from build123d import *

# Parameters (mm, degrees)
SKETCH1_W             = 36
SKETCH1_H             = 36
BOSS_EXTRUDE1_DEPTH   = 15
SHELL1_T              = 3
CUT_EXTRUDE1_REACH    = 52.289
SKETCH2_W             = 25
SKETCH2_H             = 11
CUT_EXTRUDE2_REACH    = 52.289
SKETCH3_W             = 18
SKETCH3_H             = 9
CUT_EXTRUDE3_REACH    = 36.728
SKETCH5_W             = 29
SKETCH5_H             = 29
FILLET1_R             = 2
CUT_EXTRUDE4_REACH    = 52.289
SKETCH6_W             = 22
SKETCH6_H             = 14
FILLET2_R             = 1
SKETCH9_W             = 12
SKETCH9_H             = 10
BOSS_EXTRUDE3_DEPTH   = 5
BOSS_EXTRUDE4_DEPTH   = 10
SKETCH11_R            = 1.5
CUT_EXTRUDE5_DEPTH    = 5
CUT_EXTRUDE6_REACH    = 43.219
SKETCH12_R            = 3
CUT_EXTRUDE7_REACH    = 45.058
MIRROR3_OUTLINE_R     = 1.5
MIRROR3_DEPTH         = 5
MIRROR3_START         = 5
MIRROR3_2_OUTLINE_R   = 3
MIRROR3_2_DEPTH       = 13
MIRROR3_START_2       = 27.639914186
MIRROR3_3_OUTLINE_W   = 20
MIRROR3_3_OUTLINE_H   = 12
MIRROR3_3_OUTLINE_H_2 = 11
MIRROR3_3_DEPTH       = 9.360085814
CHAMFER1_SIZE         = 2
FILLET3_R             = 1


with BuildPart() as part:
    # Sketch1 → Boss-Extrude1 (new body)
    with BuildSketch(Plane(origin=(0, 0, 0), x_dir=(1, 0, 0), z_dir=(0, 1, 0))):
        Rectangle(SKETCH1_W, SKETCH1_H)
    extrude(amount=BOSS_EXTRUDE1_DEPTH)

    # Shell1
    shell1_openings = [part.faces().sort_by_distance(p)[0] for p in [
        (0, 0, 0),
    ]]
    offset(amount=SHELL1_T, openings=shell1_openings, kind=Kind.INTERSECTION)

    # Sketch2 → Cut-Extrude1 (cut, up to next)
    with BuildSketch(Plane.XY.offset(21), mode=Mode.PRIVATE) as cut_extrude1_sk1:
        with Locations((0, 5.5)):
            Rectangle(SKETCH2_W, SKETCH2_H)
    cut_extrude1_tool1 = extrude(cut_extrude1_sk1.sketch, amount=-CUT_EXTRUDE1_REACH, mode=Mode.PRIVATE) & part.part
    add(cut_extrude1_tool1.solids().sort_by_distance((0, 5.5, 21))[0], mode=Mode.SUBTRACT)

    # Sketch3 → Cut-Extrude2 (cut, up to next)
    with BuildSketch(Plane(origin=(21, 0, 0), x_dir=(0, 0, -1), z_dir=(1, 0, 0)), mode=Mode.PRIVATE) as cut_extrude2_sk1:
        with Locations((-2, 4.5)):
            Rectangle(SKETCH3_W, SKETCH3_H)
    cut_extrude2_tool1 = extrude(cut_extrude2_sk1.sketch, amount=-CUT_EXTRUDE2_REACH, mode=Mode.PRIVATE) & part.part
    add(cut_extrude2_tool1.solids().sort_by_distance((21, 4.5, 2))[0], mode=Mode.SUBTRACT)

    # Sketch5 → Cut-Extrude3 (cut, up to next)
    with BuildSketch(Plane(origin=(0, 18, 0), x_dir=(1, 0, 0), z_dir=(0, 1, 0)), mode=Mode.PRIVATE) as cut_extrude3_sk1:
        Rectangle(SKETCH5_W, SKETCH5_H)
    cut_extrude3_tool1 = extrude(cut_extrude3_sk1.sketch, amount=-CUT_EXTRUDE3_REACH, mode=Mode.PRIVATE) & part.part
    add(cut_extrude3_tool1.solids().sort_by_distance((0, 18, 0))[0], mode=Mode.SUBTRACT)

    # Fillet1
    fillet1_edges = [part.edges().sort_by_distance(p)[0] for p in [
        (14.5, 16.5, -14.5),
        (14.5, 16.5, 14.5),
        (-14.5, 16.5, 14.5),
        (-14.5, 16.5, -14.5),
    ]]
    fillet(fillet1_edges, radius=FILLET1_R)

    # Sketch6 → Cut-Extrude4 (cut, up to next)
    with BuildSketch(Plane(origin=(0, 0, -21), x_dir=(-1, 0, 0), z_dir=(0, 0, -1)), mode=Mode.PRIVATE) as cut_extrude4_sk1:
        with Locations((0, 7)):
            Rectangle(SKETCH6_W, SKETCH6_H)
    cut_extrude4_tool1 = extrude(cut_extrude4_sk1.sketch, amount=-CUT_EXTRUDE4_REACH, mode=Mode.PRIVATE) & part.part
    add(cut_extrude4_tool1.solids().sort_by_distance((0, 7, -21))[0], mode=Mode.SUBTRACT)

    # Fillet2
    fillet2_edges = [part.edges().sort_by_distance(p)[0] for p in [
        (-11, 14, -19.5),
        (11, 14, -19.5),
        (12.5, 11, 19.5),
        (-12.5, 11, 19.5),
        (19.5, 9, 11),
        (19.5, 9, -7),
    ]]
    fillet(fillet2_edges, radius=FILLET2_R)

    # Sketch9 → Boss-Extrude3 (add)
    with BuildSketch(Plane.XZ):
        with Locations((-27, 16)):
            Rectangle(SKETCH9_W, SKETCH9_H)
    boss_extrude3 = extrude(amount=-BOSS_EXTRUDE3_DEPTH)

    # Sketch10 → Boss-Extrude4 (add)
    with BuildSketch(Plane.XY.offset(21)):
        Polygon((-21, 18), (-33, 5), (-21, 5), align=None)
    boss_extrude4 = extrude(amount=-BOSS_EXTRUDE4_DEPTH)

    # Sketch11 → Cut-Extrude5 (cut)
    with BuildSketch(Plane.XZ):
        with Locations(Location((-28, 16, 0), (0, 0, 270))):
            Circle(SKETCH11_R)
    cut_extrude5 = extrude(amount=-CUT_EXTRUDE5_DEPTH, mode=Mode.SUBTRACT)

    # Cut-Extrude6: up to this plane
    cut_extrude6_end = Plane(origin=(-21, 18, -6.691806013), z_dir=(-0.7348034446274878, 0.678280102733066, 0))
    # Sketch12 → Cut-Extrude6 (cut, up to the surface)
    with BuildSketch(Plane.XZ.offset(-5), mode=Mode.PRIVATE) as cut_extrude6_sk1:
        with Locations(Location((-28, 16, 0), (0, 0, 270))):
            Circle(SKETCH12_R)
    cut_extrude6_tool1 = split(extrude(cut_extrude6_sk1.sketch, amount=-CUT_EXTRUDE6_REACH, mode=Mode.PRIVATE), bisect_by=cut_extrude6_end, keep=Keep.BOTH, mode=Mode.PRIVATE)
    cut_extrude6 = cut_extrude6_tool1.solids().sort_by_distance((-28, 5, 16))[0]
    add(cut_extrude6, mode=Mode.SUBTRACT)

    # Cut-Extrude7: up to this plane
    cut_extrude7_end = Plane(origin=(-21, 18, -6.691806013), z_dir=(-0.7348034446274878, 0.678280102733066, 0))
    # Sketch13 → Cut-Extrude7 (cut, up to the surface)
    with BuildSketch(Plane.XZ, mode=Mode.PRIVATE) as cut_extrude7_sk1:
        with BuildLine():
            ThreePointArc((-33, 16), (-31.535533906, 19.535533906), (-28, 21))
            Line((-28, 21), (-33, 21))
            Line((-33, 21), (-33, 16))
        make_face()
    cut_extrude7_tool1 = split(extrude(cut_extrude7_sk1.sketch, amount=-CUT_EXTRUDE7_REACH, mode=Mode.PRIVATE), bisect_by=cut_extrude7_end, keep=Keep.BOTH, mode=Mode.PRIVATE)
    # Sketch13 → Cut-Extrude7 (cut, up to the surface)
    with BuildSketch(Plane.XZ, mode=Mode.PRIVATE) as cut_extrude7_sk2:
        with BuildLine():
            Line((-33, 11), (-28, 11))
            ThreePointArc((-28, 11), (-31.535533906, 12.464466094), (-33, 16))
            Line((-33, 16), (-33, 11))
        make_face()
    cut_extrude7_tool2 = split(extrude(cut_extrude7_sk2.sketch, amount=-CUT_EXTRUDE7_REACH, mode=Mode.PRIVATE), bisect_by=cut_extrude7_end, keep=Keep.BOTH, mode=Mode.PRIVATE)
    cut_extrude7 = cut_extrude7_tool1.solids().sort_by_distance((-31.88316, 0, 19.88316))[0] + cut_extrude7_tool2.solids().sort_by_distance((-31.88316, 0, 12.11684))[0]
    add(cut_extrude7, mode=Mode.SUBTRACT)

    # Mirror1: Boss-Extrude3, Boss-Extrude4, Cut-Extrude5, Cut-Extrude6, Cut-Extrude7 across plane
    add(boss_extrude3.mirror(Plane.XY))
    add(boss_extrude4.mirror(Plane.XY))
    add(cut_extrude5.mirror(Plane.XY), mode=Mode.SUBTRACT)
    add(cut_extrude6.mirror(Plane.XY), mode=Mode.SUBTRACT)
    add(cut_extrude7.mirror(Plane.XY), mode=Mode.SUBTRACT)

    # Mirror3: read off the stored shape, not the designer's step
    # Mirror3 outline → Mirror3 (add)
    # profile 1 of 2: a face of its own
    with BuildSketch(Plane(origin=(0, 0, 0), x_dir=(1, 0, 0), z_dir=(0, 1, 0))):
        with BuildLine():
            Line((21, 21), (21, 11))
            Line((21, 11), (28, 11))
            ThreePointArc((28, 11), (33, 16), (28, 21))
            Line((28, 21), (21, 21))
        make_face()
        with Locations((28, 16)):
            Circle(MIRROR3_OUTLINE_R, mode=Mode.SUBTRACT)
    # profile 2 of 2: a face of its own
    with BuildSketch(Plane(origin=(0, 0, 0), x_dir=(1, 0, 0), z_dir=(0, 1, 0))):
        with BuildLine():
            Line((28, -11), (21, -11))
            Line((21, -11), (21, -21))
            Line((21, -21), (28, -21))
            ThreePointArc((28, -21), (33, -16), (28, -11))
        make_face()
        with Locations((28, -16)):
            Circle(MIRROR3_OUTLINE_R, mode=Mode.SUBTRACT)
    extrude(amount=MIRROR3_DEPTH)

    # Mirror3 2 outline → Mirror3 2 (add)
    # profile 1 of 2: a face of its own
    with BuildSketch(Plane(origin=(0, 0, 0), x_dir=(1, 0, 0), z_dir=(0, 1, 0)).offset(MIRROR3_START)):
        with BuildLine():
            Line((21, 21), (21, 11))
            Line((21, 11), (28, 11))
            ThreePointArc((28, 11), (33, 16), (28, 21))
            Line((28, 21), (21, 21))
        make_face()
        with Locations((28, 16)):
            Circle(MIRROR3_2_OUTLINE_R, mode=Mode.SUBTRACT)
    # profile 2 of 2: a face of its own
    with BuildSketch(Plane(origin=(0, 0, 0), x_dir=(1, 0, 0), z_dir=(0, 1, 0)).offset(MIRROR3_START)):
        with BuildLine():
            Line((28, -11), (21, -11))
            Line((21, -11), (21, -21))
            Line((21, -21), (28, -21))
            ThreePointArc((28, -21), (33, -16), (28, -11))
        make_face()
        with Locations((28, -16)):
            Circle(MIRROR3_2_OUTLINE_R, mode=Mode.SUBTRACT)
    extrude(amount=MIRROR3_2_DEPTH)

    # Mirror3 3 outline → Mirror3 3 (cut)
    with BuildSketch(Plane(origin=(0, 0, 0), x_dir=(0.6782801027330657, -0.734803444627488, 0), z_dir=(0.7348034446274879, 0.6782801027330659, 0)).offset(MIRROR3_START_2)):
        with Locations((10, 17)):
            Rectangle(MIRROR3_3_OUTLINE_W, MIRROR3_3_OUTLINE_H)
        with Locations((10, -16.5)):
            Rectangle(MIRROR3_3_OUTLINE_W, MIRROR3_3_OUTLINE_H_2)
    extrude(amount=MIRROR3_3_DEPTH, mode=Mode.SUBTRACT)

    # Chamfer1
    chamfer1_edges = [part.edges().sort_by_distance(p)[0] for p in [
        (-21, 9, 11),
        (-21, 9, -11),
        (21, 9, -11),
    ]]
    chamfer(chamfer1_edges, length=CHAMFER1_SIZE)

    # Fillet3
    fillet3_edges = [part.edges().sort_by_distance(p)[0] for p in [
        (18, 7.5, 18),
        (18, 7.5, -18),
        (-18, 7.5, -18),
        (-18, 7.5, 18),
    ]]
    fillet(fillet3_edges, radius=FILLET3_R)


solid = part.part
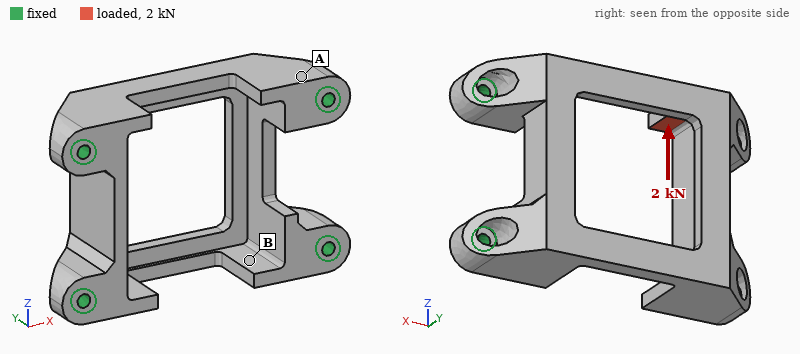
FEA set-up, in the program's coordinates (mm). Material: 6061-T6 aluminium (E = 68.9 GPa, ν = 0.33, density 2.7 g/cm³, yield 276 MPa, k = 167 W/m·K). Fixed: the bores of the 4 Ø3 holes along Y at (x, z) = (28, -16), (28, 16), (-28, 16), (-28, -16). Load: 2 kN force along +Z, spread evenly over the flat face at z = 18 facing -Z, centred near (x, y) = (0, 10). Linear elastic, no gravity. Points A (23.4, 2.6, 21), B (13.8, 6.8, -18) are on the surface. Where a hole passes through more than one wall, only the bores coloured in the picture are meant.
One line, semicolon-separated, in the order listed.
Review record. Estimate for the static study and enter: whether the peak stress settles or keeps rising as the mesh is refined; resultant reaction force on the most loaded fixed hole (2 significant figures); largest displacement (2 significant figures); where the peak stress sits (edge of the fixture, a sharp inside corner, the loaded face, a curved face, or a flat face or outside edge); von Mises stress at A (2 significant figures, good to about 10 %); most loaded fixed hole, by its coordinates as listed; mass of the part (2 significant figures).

keeps rising; 680 N; 97 µm; edge of the fixture; 36 MPa; (-28, -16); 33 g
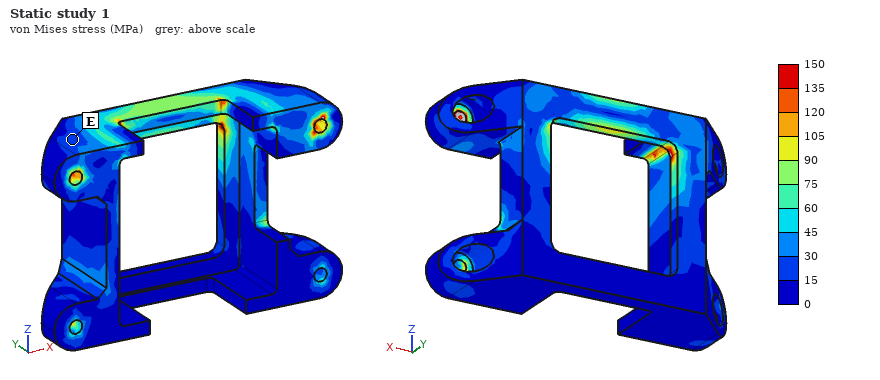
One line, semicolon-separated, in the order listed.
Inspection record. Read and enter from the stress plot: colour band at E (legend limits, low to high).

15 to 30 MPa
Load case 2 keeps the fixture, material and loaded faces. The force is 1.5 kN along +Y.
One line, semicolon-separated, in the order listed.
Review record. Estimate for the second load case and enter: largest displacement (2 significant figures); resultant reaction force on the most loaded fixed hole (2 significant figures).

35 µm; 1.1 kN
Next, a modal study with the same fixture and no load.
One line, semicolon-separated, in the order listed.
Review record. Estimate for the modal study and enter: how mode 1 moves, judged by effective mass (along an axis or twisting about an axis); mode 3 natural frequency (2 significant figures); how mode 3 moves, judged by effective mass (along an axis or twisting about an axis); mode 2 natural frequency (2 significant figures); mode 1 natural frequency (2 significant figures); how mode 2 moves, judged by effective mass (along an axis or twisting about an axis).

along X; 13 kHz; along Y; 11 kHz; 10 kHz; along Z
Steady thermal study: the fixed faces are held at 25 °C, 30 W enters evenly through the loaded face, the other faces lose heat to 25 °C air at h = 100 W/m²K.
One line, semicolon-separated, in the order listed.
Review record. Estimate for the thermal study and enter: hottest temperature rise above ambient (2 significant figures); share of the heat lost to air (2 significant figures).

26 K; 13 %
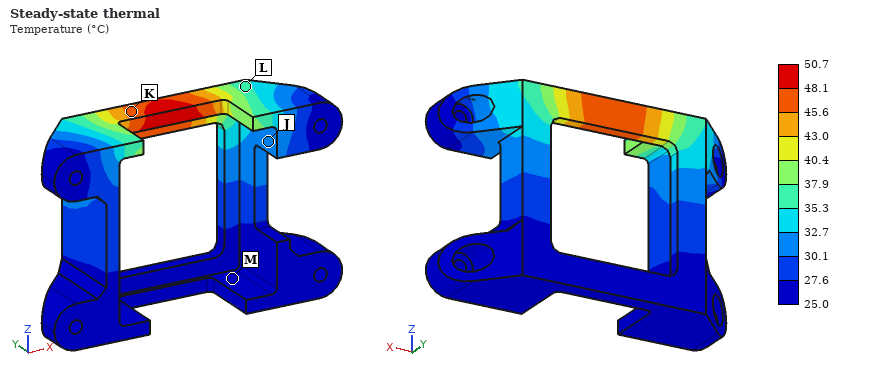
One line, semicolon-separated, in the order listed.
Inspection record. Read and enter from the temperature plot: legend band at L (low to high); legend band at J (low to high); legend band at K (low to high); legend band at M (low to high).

35.3 to 37.9 °C; 30.1 to 32.7 °C; 45.6 to 48.1 °C; 25.0 to 27.6 °C
